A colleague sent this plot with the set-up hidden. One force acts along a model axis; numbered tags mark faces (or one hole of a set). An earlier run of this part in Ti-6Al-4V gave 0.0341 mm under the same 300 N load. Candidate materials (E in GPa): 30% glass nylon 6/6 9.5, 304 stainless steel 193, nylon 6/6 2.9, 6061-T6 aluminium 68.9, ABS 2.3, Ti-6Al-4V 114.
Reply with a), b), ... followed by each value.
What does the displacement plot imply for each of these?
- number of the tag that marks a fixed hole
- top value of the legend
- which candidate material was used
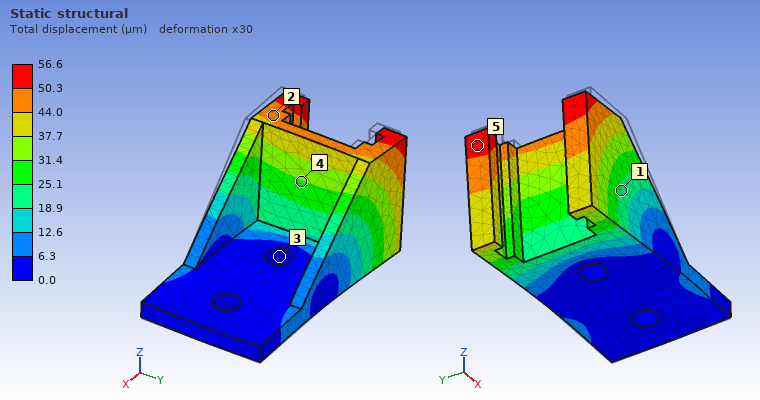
a) 3
b) 56.6 µm
c) 6061-T6 aluminium
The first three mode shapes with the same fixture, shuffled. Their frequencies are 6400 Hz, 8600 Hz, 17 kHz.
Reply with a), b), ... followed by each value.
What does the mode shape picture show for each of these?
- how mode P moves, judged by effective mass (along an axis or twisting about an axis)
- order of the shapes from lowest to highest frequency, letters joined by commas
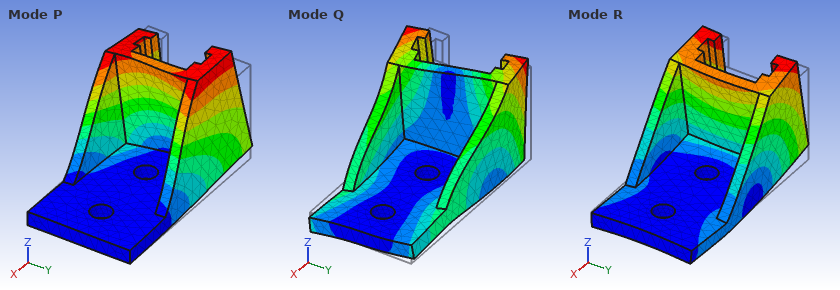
a) along Y
b) P, R, Q
